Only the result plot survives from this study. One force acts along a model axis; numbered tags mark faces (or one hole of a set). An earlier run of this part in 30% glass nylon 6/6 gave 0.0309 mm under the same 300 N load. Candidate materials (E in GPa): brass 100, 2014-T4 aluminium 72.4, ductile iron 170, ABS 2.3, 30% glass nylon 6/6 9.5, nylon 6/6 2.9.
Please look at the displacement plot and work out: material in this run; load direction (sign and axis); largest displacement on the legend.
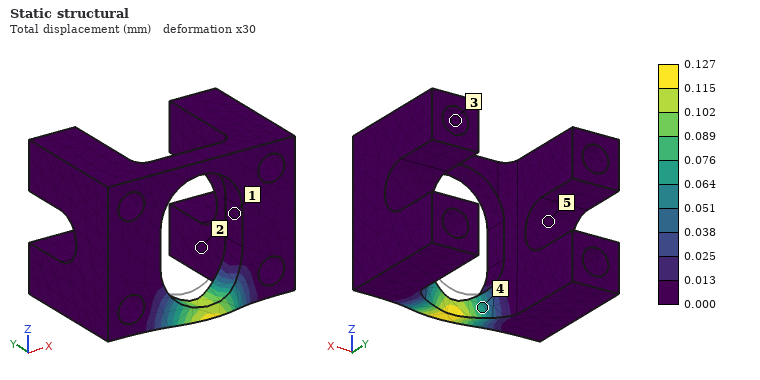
ABS
-Y
0.127 mm
